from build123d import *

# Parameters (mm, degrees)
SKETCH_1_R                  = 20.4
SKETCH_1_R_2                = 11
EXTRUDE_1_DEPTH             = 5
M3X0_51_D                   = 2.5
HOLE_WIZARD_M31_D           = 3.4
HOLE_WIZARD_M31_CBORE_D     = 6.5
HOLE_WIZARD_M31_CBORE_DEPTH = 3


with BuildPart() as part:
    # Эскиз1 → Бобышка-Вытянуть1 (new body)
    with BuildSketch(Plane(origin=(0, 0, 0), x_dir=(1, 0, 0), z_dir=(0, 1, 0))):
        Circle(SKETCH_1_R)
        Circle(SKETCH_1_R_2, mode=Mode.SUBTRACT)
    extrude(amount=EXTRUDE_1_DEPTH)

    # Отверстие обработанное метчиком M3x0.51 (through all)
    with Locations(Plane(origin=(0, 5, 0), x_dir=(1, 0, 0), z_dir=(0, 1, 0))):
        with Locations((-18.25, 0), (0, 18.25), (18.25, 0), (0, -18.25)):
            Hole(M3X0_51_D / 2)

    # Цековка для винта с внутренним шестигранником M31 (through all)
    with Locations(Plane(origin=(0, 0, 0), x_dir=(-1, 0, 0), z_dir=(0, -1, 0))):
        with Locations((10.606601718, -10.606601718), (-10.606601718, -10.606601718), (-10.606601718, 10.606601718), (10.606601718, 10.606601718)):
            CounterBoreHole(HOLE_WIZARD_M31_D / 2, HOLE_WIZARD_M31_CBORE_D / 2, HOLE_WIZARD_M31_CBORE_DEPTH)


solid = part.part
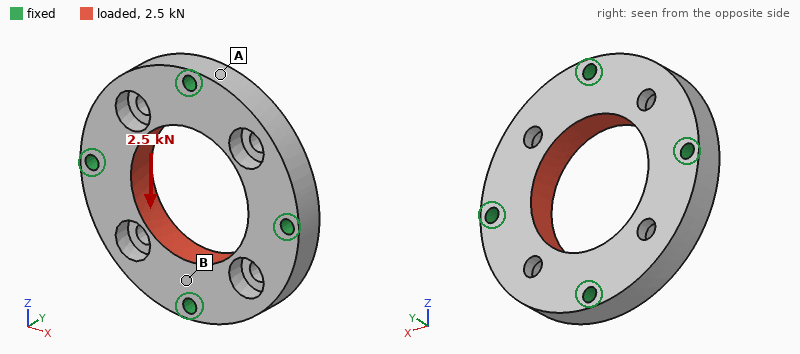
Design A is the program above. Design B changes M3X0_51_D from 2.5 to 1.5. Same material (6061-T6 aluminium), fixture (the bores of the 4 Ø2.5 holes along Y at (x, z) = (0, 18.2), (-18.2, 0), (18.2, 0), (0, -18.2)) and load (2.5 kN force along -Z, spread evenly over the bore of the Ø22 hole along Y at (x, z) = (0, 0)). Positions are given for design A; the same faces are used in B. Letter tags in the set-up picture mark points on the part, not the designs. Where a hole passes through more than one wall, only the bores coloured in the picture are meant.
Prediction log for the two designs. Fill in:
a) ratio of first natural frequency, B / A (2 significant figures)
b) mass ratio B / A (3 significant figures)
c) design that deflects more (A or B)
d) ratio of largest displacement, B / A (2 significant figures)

0.87
1.02
B
1.1
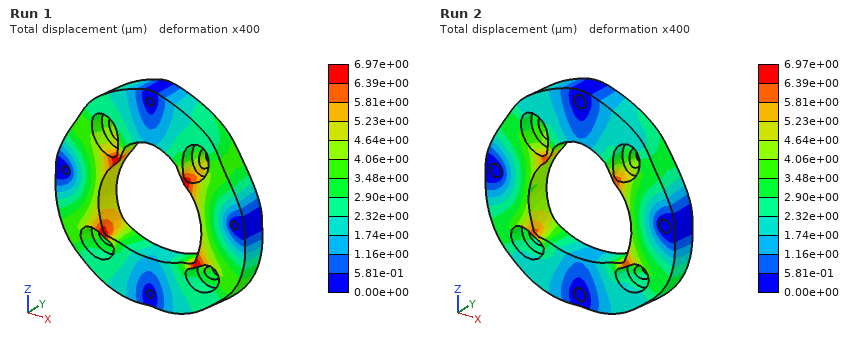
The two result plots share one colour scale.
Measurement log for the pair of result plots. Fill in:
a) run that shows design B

Run 1
